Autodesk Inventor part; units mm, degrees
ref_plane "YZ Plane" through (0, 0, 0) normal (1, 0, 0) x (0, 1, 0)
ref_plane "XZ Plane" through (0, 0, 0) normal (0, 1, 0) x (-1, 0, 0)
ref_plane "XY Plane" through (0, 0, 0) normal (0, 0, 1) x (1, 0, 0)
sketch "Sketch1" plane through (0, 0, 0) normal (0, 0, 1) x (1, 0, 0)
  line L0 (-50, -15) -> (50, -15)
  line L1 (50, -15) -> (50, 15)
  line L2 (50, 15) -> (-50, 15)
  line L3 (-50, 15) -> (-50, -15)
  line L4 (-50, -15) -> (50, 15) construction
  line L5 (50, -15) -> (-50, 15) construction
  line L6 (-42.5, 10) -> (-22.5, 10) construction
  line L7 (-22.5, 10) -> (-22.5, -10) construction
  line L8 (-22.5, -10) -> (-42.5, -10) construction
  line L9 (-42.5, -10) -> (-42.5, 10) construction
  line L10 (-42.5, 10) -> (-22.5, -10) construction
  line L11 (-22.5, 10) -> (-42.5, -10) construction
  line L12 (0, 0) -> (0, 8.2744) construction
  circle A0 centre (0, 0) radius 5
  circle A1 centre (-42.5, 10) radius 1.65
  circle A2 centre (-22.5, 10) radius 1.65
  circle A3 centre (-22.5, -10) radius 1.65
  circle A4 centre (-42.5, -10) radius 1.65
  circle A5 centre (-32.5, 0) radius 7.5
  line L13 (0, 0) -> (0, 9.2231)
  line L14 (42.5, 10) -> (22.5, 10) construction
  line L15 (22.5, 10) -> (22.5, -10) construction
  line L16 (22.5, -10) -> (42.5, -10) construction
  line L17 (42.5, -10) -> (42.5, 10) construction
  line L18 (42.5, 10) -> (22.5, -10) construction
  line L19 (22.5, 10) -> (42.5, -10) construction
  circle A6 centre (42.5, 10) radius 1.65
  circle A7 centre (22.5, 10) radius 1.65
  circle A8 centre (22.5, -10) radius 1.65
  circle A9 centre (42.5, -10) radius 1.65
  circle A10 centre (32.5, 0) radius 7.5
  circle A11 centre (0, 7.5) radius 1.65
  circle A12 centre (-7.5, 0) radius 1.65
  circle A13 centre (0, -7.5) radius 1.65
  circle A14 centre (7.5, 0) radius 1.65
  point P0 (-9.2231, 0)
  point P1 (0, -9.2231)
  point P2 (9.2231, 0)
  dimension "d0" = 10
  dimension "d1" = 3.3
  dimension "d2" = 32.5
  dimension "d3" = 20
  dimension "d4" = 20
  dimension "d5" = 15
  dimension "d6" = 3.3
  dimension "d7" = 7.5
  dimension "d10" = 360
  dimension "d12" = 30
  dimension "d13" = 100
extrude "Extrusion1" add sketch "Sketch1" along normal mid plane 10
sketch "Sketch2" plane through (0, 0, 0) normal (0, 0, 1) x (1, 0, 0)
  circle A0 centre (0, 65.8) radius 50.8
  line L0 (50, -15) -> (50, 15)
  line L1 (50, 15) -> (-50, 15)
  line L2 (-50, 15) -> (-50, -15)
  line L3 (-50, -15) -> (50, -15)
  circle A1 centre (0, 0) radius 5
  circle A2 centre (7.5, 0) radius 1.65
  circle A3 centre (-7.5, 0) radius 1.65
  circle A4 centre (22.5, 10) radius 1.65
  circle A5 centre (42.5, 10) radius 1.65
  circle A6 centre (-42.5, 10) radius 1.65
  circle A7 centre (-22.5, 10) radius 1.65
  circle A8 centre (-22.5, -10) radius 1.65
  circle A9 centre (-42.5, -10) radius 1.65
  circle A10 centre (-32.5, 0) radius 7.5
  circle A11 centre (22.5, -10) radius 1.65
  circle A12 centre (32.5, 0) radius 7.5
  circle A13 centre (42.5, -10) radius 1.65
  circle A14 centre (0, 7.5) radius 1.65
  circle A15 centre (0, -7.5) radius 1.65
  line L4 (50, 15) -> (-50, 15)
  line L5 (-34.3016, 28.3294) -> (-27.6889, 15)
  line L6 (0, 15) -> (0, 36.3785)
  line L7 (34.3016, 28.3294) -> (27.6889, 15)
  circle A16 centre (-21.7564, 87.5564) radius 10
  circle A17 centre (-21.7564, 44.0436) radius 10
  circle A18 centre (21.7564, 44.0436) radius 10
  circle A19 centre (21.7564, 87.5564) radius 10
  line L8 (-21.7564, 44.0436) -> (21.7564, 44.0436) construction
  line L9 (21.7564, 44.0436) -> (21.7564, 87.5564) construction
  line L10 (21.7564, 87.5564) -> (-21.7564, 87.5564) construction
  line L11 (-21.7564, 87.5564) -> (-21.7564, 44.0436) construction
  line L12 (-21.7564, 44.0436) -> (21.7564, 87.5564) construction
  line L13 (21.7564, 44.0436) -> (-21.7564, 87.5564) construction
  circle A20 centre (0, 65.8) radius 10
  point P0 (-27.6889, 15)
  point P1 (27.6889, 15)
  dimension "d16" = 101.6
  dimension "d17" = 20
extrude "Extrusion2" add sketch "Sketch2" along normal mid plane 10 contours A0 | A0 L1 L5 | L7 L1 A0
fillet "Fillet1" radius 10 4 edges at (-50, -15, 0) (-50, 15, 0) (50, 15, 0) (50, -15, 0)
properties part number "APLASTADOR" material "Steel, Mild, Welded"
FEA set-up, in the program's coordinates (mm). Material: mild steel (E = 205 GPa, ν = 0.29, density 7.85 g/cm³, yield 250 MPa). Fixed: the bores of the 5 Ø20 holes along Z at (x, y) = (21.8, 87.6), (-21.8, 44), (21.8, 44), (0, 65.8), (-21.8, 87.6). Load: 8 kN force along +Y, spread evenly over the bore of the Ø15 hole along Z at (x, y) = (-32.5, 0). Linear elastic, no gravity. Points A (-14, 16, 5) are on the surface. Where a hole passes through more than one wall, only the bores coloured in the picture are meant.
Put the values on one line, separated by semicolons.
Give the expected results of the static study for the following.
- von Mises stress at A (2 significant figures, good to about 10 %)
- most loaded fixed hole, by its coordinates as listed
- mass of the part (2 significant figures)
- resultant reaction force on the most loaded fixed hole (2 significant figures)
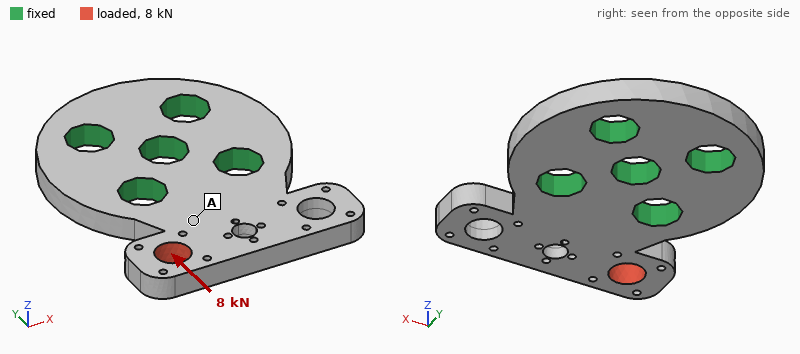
22 MPa; (-21.8, 44); 720 g; 9.0 kN
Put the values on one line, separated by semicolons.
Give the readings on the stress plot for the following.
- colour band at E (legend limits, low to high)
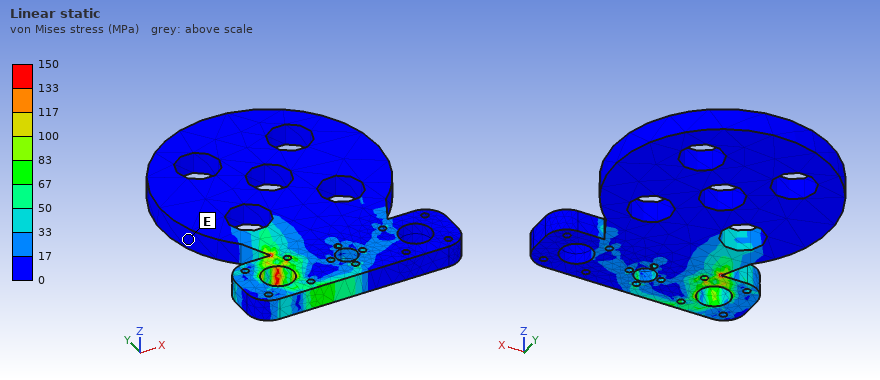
0 to 17 MPa
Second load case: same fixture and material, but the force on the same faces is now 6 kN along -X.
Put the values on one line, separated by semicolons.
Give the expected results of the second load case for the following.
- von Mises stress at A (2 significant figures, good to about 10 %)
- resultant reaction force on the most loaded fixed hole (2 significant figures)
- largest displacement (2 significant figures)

21 MPa; 5.2 kN; 17 µm
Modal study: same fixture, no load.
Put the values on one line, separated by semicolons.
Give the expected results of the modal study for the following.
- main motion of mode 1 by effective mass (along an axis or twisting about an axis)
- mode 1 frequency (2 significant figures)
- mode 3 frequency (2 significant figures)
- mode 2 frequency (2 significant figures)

along Z; 2700 Hz; 6100 Hz; 3400 Hz
